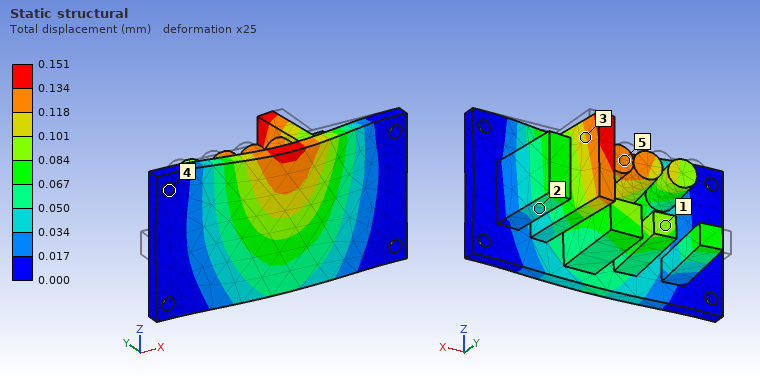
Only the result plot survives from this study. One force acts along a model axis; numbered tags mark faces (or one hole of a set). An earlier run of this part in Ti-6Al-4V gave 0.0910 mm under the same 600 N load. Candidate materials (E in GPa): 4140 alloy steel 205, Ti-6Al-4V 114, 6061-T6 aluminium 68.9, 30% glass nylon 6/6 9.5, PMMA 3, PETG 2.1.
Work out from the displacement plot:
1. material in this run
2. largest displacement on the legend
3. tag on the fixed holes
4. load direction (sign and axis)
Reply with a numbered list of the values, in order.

1. 6061-T6 aluminium
2. 0.151 mm
3. 4
4. -Y
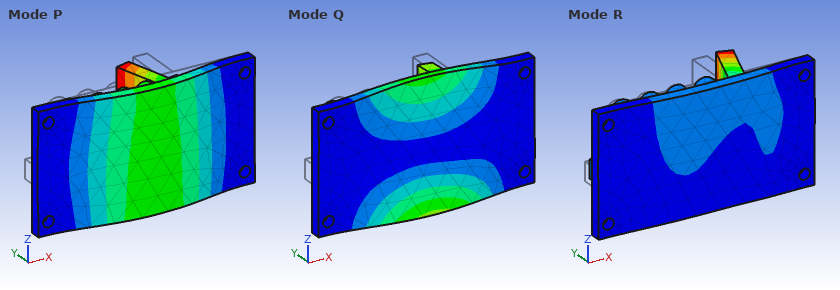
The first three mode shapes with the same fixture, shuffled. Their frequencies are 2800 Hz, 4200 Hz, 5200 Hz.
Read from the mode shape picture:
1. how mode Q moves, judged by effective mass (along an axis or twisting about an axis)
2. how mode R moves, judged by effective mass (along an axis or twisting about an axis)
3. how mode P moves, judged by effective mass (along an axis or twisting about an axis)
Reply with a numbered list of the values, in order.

1. along Z
2. along Y
3. along Y
